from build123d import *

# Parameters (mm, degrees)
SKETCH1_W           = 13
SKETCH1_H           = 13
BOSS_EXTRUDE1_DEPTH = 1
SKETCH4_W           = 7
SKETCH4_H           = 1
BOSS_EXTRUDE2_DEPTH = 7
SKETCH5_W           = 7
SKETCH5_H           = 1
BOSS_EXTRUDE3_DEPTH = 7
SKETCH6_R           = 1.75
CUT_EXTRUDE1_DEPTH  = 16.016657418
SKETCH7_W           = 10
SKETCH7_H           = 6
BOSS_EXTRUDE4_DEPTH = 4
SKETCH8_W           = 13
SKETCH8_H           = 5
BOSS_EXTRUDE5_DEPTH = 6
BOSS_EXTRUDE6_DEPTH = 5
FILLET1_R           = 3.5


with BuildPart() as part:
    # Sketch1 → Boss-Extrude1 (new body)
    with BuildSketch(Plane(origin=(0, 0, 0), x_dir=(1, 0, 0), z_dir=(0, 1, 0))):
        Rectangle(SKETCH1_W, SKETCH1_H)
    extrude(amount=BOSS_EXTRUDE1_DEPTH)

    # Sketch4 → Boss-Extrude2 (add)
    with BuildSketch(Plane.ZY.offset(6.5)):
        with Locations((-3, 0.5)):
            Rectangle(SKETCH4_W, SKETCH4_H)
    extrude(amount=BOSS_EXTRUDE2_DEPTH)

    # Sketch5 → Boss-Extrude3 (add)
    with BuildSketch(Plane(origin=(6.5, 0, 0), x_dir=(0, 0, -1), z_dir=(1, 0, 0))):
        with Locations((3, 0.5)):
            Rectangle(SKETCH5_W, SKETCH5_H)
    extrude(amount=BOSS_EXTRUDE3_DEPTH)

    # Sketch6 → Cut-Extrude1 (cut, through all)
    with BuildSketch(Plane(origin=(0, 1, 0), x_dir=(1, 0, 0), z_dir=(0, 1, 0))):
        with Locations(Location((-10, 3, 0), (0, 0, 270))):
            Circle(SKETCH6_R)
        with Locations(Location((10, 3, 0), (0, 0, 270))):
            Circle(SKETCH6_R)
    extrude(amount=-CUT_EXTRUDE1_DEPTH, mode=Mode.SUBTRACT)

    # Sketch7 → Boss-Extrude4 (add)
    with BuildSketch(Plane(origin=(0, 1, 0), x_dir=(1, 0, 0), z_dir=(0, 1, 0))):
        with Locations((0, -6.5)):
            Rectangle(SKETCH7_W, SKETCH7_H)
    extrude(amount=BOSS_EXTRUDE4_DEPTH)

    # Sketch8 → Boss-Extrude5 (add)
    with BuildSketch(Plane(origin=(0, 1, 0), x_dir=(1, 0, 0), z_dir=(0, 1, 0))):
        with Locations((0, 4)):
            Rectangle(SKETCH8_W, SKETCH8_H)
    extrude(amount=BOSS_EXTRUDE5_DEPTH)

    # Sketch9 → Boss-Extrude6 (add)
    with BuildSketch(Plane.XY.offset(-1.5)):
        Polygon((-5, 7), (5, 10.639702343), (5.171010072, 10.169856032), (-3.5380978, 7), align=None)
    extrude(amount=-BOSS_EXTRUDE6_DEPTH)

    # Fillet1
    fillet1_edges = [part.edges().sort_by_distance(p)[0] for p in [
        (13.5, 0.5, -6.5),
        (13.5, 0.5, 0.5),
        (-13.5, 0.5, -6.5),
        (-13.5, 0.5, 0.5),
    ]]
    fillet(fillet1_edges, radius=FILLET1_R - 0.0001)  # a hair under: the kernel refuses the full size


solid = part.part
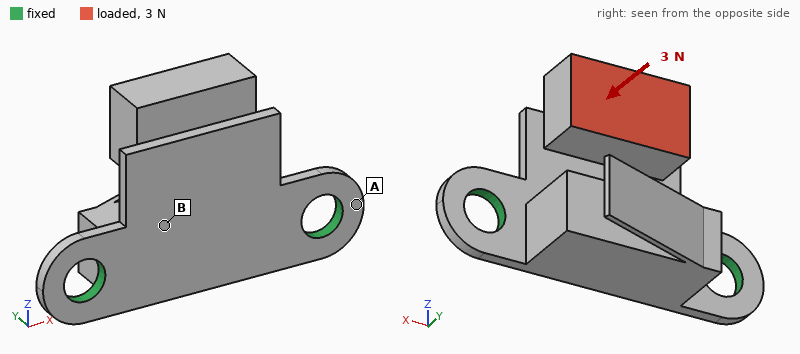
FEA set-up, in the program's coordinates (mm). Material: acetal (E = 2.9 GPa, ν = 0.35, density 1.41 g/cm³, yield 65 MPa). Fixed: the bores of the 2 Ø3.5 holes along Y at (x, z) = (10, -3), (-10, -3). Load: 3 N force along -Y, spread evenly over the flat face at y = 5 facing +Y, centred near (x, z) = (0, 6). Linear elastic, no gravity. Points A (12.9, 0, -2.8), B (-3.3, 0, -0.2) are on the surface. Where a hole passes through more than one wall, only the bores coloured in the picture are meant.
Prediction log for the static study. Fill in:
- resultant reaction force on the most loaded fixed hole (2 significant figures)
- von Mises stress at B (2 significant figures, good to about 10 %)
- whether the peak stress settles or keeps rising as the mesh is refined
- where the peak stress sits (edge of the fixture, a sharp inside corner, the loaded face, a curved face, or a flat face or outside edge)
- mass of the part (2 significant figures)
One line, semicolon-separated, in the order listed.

1.8 N; 7.0 MPa; keeps rising; a sharp inside corner; 1.3 g
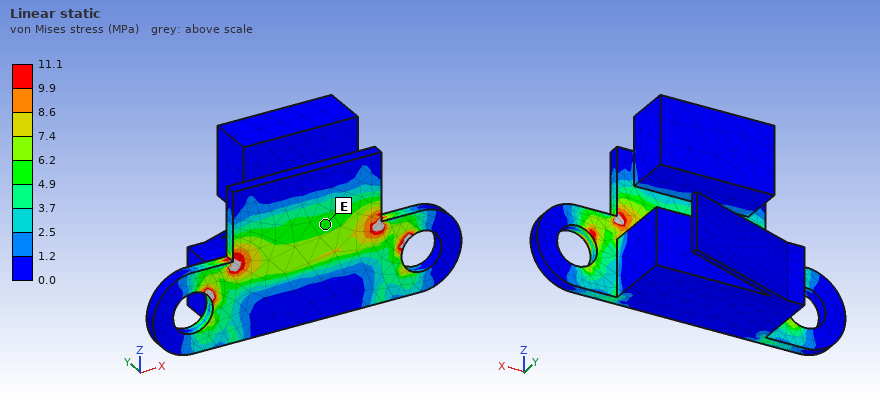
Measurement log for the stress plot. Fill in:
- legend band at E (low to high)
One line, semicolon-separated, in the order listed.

4.9 to 6.2 MPa
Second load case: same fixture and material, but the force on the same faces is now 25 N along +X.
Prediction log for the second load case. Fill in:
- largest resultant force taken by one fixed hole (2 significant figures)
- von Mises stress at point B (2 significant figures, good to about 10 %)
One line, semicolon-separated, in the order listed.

20 N; 12 MPa
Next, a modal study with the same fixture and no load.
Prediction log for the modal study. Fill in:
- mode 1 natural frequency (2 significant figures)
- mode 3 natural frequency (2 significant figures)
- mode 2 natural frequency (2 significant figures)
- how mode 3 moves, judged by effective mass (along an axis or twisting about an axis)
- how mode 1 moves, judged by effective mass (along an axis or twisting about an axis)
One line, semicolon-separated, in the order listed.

840 Hz; 2900 Hz; 1300 Hz; along Z; along Y
